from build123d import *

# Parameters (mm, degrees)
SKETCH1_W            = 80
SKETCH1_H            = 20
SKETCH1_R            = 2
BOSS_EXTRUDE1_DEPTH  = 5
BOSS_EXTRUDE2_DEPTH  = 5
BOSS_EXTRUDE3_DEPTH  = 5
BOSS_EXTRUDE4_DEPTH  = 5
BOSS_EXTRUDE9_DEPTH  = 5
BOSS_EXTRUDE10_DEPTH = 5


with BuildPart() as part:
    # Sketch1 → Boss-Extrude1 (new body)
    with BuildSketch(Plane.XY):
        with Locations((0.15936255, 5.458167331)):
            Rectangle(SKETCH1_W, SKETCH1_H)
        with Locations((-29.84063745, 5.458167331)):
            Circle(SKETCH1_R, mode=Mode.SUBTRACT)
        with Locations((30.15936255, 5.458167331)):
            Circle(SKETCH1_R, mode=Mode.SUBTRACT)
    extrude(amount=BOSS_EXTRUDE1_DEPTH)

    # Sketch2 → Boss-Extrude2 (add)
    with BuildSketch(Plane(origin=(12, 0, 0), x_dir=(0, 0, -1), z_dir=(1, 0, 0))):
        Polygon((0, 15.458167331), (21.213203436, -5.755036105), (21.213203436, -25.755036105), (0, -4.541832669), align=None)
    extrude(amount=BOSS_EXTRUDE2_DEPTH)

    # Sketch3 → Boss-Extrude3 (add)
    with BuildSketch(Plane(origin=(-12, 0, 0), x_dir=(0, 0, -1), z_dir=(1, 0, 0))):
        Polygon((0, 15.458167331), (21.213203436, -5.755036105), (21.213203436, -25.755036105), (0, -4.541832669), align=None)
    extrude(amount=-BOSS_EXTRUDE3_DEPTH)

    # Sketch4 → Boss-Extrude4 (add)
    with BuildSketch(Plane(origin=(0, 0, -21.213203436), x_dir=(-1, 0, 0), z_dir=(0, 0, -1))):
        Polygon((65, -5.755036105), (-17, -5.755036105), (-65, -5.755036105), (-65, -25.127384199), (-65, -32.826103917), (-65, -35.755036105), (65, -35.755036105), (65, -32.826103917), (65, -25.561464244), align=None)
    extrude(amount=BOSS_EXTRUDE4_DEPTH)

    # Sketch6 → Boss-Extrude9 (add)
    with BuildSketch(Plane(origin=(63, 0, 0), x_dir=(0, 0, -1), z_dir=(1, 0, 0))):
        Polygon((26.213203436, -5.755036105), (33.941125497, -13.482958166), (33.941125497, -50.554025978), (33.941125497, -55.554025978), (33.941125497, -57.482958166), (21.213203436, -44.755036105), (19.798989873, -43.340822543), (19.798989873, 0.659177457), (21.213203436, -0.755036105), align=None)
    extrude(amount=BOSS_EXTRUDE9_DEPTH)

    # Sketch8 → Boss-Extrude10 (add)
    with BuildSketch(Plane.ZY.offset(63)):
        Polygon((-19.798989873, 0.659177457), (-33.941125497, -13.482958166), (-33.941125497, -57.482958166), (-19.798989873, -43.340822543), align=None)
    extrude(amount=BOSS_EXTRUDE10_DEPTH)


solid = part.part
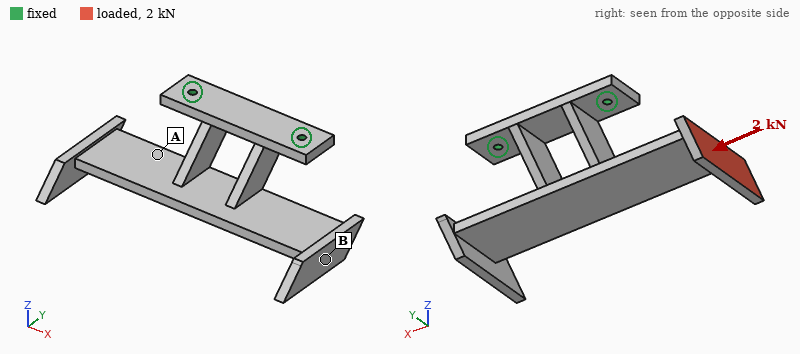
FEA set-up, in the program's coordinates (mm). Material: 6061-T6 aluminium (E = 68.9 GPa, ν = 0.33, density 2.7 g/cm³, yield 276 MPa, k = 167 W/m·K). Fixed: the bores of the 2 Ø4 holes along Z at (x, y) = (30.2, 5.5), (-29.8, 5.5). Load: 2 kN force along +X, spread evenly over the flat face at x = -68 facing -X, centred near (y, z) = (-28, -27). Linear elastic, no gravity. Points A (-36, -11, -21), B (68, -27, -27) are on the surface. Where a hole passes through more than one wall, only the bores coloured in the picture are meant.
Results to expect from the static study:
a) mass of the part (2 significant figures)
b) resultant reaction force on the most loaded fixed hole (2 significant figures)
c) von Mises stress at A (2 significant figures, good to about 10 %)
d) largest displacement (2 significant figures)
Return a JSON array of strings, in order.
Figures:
["100 g", "2.0 kN", "47 MPa", "1.0 mm"]
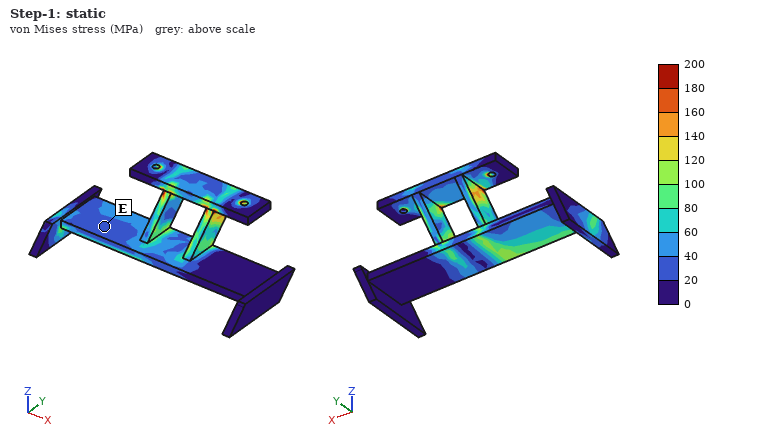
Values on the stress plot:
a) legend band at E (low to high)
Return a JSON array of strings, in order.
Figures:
["20 to 40 MPa"]
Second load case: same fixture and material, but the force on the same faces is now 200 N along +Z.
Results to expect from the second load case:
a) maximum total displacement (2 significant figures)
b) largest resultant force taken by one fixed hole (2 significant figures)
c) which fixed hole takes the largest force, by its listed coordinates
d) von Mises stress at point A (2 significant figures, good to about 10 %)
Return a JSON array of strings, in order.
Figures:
["1.2 mm", "390 N", "(-29.8, 5.5)", "51 MPa"]
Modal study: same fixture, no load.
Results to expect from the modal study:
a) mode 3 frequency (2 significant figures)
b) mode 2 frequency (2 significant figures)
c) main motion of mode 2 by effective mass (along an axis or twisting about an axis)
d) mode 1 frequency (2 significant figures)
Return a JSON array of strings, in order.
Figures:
["1100 Hz", "610 Hz", "along Z", "580 Hz"]
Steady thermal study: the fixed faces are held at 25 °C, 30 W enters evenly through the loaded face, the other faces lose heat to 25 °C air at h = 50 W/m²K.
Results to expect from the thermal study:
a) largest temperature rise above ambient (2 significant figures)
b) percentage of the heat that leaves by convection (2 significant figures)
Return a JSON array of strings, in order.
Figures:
["81 K", "62 %"]
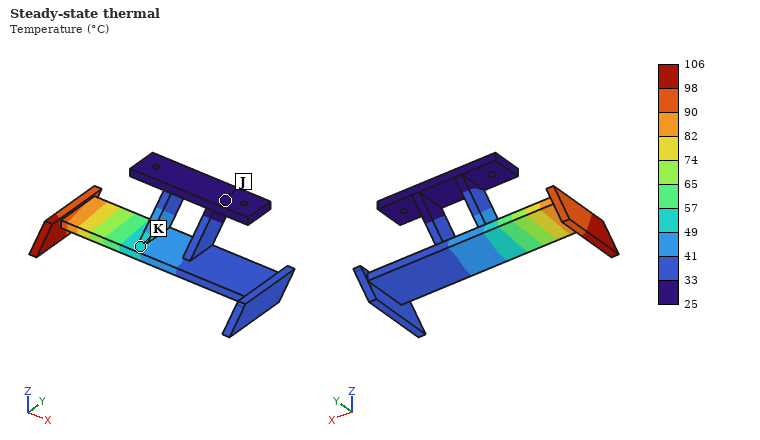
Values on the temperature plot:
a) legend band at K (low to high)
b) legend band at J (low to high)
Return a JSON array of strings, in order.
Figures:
["49 to 57 °C", "25 to 33 °C"]
